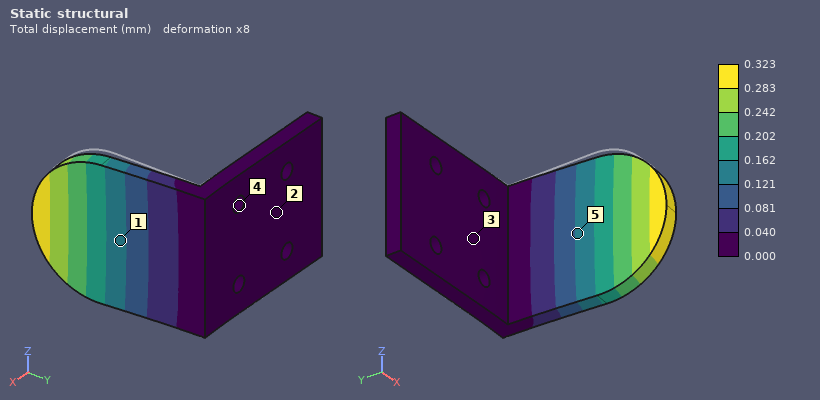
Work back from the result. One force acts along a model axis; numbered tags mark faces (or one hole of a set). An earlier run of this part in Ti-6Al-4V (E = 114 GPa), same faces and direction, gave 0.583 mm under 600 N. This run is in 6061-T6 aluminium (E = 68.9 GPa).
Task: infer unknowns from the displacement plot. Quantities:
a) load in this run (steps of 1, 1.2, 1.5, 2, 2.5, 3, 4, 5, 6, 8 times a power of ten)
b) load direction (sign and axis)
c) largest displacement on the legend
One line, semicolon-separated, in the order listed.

200 N; +X; 0.323 mm
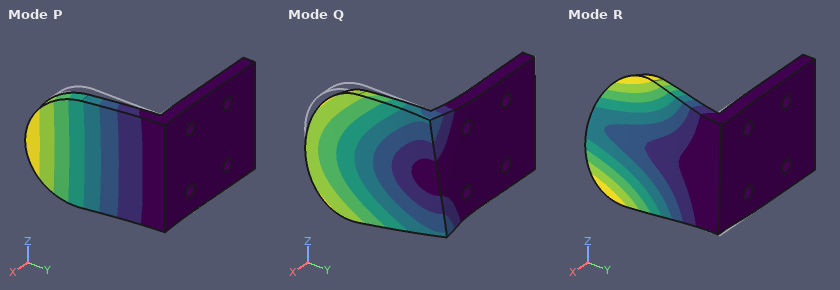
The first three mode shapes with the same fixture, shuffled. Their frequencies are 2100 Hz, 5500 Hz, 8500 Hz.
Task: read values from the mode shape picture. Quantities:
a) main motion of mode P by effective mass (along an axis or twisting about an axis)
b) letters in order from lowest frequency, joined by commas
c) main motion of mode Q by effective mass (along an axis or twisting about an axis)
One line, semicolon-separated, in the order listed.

along X; P, Q, R; along Z
